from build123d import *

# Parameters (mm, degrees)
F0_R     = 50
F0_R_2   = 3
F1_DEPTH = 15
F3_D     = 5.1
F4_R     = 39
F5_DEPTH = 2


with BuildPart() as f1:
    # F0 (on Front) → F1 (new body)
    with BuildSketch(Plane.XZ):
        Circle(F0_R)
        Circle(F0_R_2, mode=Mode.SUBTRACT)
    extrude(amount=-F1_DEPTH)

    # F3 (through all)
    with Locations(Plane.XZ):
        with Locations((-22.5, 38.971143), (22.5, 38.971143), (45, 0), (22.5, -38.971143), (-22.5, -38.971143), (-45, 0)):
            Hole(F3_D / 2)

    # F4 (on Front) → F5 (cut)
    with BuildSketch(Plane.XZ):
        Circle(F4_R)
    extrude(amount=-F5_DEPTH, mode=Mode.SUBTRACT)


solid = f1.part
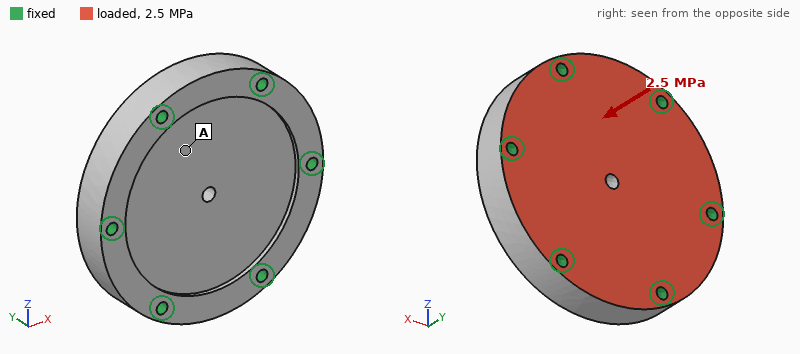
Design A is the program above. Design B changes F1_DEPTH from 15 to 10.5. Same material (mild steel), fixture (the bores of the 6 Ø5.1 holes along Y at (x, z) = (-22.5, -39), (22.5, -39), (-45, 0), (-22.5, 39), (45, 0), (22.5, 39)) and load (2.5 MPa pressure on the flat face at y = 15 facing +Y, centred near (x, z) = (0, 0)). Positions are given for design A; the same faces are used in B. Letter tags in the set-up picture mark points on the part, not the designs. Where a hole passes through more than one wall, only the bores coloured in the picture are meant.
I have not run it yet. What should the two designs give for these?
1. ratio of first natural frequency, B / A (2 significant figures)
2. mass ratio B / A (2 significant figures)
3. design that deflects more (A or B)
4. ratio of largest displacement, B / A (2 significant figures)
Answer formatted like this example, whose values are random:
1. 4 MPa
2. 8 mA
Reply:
1. 0.76
2. 0.67
3. B
4. 2.7
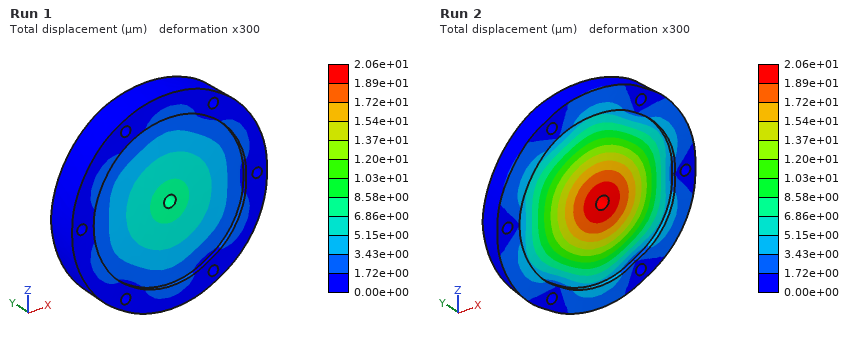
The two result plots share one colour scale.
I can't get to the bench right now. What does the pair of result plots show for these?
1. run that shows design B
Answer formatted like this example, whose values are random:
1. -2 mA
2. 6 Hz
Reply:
1. Run 2
